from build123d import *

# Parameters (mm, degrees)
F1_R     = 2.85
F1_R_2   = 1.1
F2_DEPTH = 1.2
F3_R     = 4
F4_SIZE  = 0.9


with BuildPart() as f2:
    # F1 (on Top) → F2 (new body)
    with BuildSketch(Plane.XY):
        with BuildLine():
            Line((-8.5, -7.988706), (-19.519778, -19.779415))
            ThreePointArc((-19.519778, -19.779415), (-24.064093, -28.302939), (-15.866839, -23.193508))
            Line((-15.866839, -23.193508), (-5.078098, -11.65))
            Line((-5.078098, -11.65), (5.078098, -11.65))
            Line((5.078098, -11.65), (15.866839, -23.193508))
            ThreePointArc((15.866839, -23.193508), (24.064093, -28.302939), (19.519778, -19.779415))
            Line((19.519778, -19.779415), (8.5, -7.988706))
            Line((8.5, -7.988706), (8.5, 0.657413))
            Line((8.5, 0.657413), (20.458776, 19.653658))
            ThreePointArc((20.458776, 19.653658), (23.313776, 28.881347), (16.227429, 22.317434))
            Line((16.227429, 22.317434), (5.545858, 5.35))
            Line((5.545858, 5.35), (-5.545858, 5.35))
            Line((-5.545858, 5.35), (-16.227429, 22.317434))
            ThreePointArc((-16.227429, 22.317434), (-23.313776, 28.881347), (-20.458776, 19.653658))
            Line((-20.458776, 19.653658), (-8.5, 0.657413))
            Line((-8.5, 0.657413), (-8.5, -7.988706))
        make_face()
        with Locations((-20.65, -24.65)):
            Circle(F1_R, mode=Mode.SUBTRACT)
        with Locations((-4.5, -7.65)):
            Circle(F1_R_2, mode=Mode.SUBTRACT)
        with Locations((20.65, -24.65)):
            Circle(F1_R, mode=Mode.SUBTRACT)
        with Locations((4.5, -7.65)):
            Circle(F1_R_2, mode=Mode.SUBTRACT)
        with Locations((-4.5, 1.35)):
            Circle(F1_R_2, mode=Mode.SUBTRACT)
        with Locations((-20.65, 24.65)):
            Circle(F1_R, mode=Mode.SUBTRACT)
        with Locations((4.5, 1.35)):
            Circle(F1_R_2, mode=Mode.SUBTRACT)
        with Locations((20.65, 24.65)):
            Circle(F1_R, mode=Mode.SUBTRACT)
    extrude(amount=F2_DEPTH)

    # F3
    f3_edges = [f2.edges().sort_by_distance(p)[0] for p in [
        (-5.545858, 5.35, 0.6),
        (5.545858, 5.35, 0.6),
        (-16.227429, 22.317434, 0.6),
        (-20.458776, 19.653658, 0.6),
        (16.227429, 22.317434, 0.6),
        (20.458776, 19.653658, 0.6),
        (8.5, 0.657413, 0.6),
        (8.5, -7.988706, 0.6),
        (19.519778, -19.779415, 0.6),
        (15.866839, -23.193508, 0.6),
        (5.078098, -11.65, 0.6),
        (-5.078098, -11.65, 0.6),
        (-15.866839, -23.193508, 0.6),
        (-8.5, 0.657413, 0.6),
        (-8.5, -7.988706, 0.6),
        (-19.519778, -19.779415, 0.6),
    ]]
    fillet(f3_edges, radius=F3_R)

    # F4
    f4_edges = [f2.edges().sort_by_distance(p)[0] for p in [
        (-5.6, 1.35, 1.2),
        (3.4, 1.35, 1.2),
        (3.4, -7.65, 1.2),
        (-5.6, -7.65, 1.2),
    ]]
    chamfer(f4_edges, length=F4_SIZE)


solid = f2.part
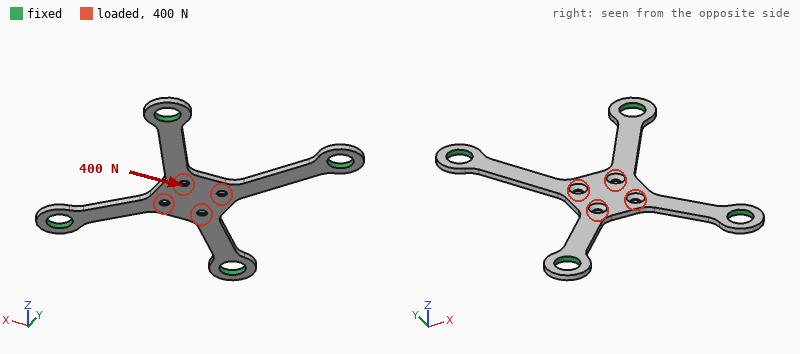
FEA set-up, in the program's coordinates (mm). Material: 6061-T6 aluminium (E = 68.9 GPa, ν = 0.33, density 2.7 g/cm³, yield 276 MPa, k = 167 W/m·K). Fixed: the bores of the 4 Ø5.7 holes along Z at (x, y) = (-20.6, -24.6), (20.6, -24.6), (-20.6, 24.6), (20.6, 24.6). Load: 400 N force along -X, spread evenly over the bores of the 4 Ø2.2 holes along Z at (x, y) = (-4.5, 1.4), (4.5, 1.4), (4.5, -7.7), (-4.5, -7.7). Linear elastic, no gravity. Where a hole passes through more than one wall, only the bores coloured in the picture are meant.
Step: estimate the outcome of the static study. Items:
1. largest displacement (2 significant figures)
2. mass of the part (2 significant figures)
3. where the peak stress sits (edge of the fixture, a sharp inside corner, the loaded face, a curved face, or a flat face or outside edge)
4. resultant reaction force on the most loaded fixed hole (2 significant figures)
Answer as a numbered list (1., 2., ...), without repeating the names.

1. 42 µm
2. 2.6 g
3. the loaded face
4. 180 N
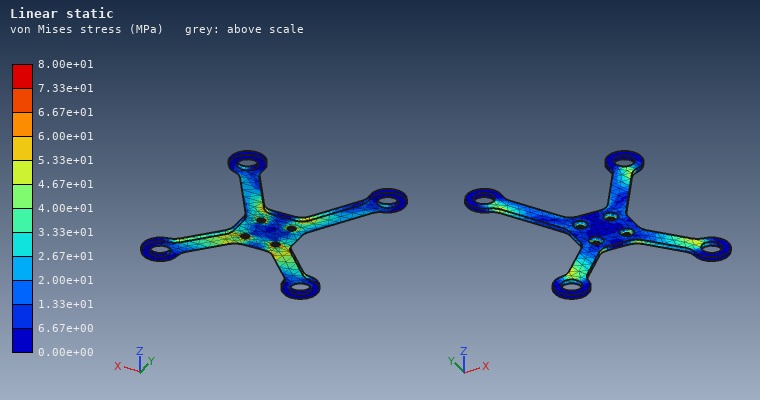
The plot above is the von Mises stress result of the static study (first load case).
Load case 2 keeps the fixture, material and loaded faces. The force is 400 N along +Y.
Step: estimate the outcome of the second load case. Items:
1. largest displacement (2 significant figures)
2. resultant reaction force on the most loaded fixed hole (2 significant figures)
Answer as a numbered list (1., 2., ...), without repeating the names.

1. 44 µm
2. 130 N
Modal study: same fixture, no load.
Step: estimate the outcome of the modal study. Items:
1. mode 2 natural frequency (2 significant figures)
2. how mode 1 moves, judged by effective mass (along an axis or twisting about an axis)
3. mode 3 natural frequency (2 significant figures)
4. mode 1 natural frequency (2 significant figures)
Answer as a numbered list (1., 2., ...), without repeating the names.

1. 4700 Hz
2. along Z
3. 5300 Hz
4. 2000 Hz
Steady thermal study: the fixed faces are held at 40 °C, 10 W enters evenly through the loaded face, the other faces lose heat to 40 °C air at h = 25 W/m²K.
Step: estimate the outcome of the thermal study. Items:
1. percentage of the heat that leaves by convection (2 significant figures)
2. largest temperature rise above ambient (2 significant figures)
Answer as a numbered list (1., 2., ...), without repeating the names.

1. 12 %
2. 54 K
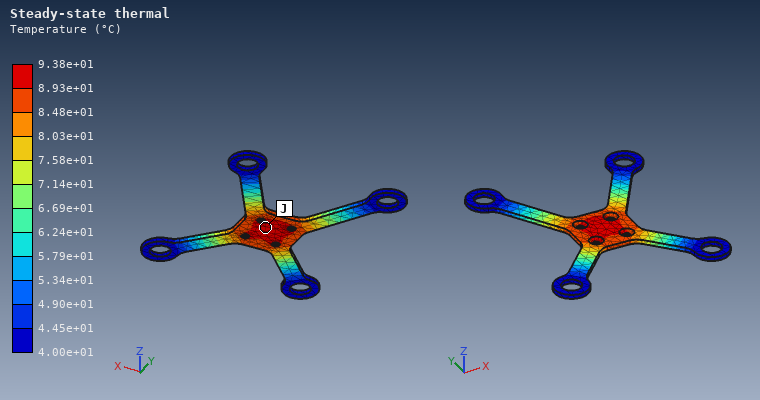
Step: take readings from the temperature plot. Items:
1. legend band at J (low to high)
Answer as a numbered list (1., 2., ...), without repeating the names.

1. 8.93e+01 to 9.38e+01 °C
